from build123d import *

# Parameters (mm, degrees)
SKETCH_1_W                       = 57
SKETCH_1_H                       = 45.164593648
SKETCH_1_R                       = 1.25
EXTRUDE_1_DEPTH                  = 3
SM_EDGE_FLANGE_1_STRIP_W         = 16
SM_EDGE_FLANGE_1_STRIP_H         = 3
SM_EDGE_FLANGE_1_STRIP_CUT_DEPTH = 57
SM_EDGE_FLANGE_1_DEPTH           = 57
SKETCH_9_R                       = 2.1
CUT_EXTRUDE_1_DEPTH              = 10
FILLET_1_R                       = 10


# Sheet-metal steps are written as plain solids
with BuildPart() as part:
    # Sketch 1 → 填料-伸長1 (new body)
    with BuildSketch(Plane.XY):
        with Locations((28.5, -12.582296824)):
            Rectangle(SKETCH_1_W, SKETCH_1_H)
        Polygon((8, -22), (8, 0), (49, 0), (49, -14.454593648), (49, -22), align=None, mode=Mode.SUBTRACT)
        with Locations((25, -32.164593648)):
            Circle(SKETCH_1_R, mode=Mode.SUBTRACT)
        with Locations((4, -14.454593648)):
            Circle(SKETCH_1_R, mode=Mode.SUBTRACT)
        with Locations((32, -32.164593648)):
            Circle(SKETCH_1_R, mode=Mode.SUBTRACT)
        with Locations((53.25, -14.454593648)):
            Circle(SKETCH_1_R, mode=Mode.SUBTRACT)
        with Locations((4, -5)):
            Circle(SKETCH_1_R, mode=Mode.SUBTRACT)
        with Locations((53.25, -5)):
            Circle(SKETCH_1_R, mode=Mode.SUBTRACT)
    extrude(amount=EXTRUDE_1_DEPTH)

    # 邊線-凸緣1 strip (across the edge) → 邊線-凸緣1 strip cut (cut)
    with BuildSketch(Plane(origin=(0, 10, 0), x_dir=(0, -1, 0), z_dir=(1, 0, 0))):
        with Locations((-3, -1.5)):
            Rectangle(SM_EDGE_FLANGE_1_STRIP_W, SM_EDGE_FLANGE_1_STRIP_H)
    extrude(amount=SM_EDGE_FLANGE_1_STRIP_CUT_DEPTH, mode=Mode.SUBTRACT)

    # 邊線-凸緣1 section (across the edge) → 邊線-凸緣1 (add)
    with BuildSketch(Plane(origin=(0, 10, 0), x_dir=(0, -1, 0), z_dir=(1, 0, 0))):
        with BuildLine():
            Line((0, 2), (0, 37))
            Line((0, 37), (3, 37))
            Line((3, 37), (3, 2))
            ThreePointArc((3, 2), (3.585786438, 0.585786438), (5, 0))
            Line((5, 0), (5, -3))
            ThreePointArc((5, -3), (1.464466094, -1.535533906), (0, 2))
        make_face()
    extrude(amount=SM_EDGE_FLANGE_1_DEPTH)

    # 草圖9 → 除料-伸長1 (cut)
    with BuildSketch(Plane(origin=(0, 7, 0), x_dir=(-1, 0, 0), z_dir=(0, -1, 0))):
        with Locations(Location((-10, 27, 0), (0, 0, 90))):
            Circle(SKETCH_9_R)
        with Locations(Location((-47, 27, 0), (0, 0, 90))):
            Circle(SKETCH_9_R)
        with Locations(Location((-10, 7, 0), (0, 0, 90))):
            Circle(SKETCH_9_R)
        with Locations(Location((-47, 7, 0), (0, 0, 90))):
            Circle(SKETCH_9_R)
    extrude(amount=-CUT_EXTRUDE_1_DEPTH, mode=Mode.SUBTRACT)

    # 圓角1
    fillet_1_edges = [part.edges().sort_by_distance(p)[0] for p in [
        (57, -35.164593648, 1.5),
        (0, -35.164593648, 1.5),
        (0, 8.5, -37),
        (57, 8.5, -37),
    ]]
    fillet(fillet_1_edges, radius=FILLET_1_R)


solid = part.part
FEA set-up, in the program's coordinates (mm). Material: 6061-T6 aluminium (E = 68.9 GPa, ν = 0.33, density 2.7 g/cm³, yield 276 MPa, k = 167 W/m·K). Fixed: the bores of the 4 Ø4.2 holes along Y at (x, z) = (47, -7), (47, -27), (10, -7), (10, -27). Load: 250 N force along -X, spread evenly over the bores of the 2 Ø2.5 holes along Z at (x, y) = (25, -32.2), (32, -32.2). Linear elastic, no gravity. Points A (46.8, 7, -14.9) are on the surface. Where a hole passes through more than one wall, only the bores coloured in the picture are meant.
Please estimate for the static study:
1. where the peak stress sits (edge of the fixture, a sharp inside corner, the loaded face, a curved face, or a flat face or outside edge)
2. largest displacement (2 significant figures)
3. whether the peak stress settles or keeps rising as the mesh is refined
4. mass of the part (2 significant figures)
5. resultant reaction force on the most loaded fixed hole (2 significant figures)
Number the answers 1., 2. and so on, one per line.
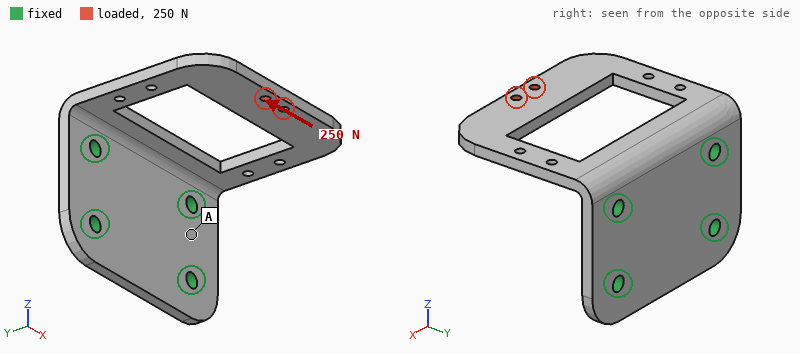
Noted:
1. edge of the fixture
2. 0.11 mm
3. keeps rising
4. 29 g
5. 290 N
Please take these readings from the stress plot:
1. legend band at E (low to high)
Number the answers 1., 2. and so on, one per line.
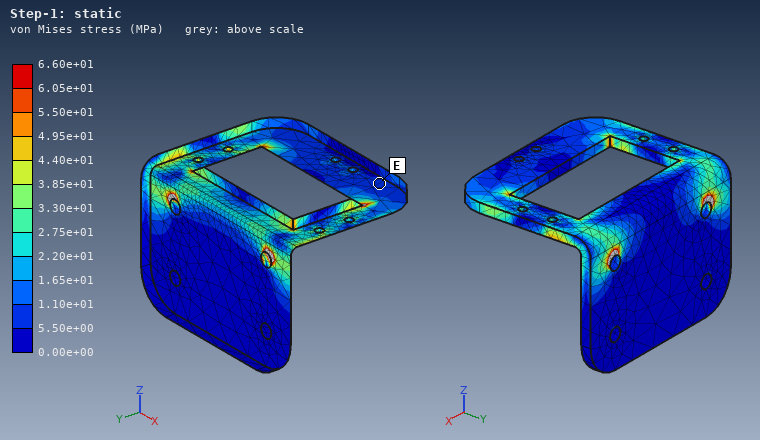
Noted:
1. 5.50e+00 to 1.10e+01 MPa
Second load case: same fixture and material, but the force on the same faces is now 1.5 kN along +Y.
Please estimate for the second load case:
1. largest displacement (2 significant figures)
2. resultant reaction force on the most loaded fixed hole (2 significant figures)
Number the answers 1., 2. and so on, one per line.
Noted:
1. 0.37 mm
2. 870 N
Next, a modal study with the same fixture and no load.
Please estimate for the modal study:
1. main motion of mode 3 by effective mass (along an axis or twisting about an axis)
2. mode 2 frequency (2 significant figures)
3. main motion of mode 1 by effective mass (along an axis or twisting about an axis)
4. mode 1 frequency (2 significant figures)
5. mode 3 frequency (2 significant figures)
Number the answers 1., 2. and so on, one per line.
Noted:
1. along X
2. 1900 Hz
3. along Z
4. 740 Hz
5. 3300 Hz
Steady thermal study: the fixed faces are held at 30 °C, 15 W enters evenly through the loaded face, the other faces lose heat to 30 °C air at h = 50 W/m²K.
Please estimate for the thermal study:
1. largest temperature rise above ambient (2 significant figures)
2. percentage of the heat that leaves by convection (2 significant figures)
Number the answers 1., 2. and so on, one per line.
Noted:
1. 68 K
2. 42 %
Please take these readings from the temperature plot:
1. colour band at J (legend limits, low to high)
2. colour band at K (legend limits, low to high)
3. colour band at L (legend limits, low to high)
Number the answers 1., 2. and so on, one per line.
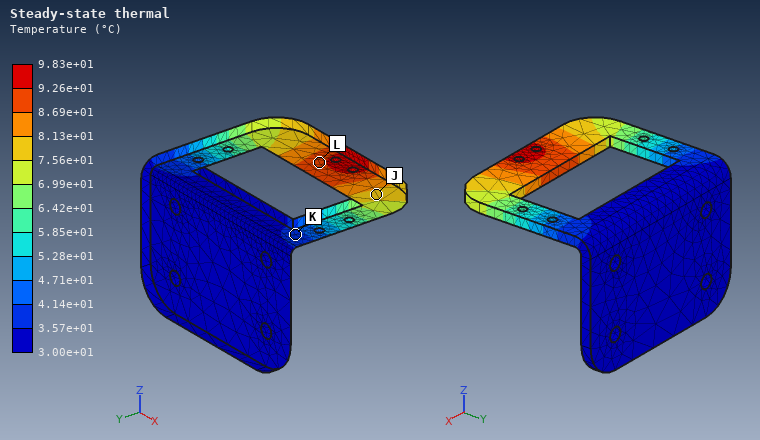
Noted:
1. 7.56e+01 to 8.13e+01 °C
2. 3.57e+01 to 4.14e+01 °C
3. 8.69e+01 to 9.26e+01 °C
